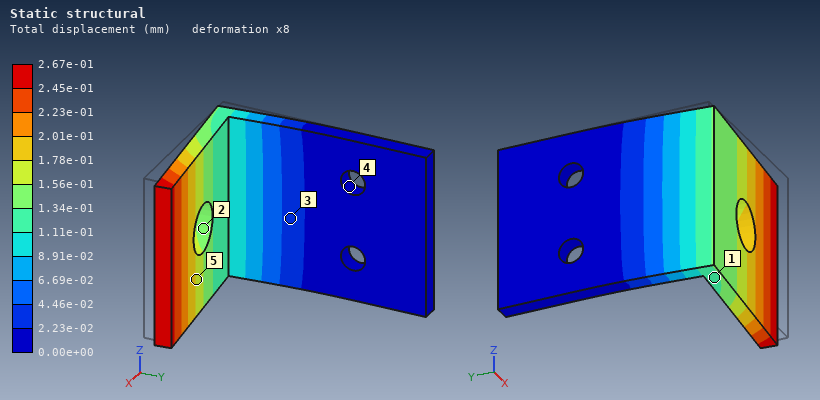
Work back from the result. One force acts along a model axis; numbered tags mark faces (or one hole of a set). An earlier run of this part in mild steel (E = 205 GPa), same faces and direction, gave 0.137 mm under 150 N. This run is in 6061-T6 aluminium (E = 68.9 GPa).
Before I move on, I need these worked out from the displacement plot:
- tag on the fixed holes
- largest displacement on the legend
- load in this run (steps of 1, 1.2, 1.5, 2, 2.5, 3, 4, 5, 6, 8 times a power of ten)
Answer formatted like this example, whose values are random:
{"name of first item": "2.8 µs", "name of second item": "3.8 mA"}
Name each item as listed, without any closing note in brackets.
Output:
{"tag on the fixed holes": "4", "largest displacement on the legend": "2.67e-01 mm", "load in this run": "100 N"}
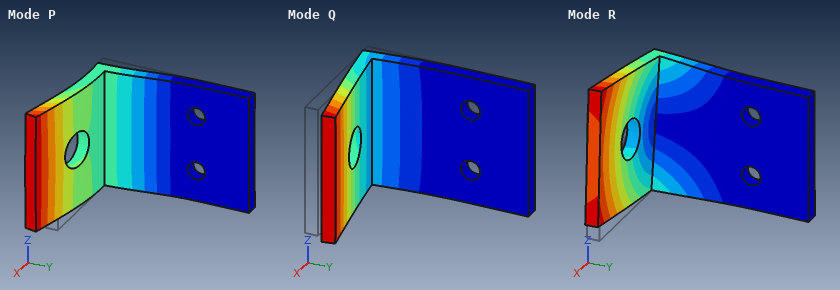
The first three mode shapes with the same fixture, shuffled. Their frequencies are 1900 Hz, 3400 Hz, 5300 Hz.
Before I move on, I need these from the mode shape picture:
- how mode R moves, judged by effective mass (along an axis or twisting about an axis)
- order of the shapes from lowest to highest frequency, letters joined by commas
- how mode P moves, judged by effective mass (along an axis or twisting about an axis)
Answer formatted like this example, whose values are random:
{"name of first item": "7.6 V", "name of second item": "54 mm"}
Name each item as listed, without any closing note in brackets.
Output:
{"how mode R moves, judged by effective mass": "along Z", "order of the shapes from lowest to highest frequency, letters joined by commas": "Q, R, P", "how mode P moves, judged by effective mass": "along X"}
